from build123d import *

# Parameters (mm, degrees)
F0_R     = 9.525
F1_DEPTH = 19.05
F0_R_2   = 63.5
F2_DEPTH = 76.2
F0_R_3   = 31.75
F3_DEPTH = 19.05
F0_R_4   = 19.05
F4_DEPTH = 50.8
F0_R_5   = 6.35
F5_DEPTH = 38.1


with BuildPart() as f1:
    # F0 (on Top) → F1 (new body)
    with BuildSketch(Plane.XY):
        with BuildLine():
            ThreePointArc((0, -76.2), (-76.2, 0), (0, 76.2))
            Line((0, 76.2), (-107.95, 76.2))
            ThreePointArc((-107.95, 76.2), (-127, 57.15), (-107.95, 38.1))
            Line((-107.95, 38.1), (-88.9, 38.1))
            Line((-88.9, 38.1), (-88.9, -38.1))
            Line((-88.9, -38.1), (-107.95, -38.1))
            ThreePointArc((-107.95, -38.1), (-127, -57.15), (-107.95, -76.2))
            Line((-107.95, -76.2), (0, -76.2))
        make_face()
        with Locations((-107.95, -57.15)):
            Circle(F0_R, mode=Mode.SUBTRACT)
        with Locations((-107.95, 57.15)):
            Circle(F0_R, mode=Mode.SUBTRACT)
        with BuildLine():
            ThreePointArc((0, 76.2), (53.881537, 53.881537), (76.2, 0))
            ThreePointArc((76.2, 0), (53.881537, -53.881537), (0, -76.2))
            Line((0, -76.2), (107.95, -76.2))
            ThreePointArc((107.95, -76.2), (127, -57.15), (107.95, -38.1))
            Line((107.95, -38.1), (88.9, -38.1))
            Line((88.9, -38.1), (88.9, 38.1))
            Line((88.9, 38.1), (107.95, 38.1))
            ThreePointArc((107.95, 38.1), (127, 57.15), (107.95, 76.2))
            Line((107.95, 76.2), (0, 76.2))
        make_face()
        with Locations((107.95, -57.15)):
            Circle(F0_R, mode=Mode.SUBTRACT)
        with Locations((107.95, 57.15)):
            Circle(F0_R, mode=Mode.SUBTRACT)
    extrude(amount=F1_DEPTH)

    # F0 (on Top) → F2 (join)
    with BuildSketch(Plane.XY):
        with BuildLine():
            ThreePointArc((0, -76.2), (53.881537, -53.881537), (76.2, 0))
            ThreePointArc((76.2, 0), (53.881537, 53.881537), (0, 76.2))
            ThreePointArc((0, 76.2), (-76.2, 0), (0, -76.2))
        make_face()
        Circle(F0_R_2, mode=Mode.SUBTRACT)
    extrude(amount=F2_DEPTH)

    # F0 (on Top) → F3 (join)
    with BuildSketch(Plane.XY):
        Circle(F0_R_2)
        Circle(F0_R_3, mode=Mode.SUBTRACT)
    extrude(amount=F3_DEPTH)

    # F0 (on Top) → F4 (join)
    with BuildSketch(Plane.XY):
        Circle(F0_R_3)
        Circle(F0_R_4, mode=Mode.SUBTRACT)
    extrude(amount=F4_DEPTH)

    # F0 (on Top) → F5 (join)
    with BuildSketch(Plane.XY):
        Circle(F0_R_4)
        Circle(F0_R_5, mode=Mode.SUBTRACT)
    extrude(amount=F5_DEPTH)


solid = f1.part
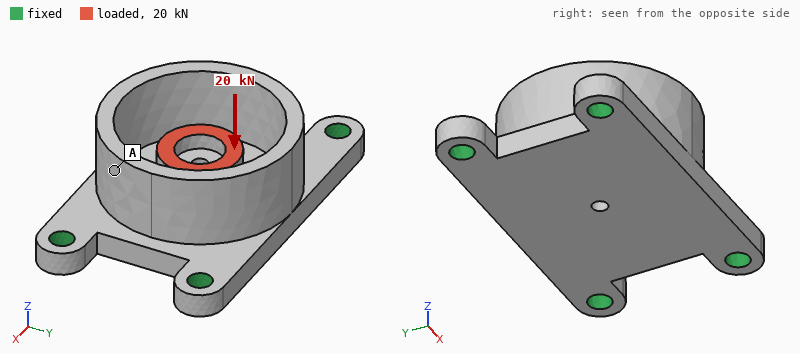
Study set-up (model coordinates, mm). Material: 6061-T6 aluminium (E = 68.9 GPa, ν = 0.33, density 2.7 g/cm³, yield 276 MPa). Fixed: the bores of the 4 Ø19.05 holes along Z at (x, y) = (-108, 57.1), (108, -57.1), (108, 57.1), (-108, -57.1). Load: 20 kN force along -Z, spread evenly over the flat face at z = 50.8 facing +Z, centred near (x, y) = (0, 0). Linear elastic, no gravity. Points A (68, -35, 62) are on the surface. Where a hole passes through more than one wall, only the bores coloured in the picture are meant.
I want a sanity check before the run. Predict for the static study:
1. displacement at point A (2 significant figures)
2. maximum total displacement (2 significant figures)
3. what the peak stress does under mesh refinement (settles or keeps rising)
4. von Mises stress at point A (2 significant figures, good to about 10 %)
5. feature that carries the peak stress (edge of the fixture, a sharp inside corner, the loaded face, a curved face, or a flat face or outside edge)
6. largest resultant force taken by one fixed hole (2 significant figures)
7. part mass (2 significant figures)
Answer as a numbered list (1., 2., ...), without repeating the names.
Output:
1. 0.060 mm
2. 0.11 mm
3. keeps rising
4. 7.5 MPa
5. edge of the fixture
6. 5.4 kN
7. 2.7 kg
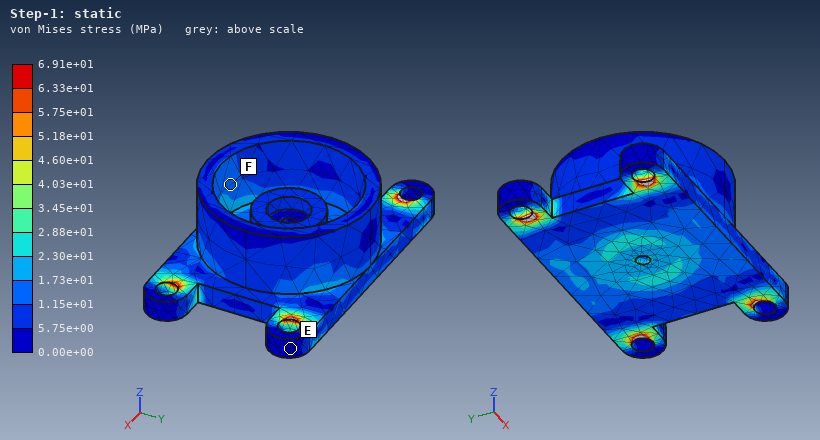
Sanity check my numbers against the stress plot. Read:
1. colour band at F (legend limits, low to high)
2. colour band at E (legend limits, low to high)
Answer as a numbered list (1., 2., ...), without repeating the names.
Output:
1. 1.15e+01 to 1.73e+01 MPa
2. 0.00e+00 to 5.75e+00 MPa
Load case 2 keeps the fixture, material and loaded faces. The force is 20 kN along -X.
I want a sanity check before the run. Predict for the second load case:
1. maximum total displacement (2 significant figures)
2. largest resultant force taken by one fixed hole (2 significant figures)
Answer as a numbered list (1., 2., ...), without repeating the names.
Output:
1. 93 µm
2. 5.9 kN
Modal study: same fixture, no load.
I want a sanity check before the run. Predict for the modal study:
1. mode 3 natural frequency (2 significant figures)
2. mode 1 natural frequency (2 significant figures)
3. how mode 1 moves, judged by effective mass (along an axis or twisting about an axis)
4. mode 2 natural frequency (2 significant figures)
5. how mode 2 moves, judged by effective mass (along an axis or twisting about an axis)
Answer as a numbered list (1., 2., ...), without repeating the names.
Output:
1. 3400 Hz
2. 1800 Hz
3. along Z
4. 2100 Hz
5. along Y
